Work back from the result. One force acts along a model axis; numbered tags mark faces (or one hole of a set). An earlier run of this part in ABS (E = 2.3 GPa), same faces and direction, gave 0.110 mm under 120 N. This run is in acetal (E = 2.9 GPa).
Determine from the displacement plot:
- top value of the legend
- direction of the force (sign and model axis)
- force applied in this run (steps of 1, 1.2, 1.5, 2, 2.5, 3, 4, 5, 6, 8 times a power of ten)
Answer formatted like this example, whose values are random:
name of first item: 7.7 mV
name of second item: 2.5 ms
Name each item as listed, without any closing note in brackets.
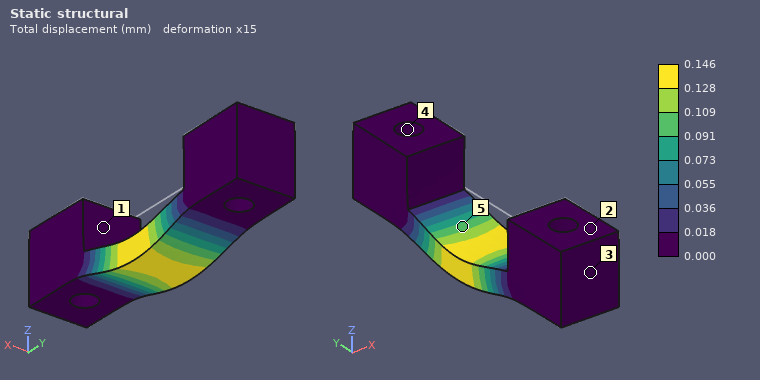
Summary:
top value of the legend: 0.146 mm
direction of the force: -Z
force applied in this run: 200 N
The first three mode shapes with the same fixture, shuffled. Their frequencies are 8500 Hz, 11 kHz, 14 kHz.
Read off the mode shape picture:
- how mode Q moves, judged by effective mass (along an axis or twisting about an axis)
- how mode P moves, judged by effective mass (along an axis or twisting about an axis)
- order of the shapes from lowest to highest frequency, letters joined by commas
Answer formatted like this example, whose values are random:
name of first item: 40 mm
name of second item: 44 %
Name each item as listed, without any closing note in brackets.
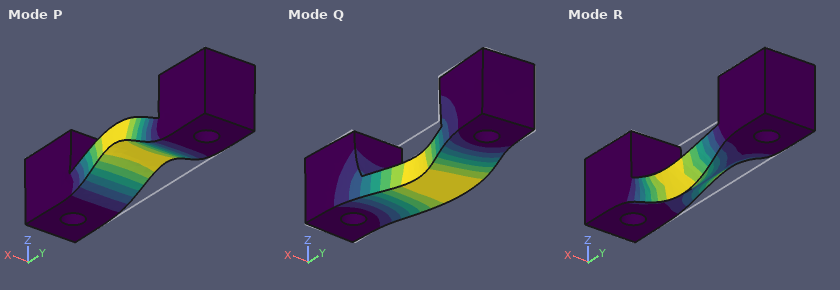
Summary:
how mode Q moves, judged by effective mass: along X
how mode P moves, judged by effective mass: along Z
order of the shapes from lowest to highest frequency, letters joined by commas: P, Q, R
